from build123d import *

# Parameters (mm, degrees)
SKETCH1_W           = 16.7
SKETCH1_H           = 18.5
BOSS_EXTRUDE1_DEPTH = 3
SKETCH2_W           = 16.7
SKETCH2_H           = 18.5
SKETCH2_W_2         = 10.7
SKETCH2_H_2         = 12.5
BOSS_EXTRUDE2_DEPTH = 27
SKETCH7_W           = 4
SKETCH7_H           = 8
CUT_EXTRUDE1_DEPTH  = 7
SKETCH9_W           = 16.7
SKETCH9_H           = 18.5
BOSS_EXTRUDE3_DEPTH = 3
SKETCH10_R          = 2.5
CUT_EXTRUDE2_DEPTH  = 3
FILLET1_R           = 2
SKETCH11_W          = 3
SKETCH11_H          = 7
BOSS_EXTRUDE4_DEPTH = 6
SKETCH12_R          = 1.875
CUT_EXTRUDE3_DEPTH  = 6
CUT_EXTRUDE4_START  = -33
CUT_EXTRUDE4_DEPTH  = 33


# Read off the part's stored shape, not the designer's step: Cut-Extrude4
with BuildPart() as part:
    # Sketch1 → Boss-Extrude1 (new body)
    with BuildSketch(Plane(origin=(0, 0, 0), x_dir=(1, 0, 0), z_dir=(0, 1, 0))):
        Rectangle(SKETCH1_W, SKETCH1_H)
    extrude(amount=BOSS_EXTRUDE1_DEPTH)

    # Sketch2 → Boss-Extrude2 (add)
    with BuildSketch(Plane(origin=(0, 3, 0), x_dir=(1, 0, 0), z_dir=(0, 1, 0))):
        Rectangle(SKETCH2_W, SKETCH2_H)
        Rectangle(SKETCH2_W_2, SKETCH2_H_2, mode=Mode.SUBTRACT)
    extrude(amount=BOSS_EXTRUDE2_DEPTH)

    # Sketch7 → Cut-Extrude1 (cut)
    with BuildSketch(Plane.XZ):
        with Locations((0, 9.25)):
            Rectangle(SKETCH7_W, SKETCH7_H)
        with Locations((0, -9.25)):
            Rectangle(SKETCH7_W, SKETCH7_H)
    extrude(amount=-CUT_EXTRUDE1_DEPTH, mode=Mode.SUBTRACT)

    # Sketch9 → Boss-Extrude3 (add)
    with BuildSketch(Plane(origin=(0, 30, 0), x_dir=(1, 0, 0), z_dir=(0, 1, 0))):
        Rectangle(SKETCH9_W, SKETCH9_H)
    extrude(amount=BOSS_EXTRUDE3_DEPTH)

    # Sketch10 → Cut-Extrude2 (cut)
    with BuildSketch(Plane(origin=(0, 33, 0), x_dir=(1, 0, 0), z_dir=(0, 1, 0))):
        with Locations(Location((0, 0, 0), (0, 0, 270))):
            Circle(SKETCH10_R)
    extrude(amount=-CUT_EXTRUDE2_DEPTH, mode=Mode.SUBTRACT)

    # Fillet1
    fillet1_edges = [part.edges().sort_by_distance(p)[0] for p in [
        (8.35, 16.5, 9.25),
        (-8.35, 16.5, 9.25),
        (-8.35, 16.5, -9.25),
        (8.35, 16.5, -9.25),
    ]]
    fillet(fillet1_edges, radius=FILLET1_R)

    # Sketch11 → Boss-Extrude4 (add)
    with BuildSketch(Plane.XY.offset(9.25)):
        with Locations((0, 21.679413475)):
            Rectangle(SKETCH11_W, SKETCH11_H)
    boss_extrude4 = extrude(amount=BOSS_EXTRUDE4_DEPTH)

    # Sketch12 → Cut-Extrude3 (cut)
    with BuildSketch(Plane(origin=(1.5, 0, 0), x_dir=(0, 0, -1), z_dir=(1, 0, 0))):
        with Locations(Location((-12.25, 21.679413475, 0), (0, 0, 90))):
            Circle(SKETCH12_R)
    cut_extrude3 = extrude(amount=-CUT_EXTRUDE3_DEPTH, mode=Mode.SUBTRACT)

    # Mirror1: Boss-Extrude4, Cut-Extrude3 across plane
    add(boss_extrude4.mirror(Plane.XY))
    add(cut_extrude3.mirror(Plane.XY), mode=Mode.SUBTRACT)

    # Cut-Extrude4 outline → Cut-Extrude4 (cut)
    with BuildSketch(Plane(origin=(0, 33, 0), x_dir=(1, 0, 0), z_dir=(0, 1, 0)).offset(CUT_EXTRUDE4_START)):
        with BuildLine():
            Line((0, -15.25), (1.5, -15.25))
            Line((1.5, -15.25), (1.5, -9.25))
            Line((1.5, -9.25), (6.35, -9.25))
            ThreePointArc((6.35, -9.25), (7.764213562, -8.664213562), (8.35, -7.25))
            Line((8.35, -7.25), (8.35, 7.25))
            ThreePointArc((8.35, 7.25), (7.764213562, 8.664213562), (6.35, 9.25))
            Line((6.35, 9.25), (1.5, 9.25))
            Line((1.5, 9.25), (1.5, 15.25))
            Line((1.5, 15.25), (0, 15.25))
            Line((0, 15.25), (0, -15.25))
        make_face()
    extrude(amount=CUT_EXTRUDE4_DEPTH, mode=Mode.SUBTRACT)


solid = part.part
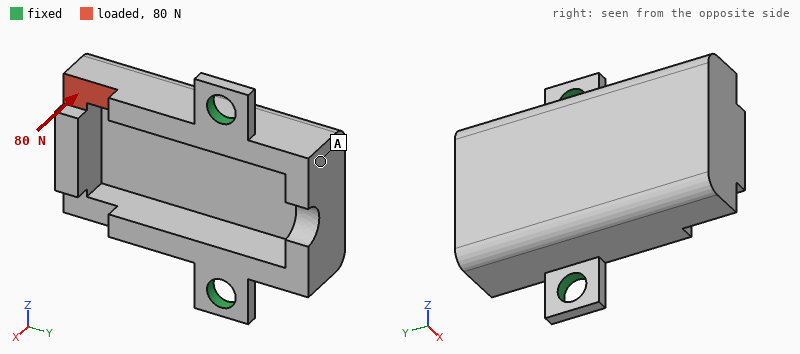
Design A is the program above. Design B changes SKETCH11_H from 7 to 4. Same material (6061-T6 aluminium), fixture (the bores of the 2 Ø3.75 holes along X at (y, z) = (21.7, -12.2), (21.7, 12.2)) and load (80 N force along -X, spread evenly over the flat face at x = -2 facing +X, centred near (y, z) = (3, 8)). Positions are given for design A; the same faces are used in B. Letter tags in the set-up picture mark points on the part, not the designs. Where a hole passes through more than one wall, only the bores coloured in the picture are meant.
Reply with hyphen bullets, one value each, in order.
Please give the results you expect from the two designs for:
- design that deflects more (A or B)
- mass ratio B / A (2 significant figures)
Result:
- B
- 0.98
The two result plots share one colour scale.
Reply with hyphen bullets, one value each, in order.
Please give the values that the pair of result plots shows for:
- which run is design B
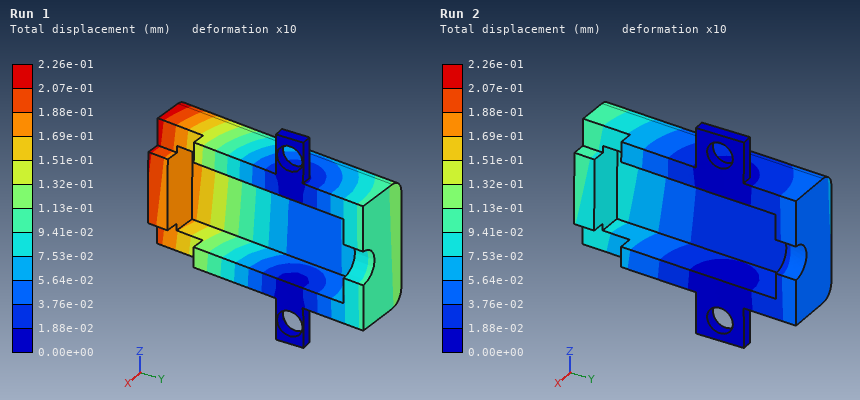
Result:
- Run 1
